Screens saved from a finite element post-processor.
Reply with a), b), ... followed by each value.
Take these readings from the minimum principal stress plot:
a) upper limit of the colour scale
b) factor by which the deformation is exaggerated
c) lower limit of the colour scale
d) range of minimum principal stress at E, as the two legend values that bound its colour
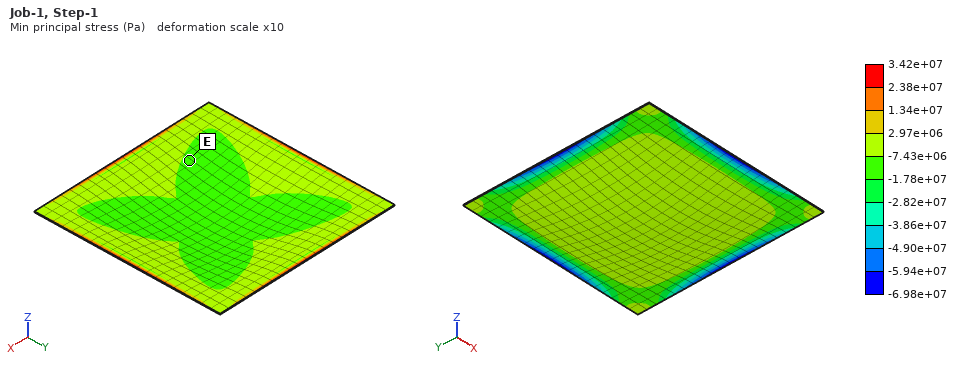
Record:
a) 3.42e+07 Pa
b) 10
c) -6.98e+07 Pa
d) -1.78e+07 to -7.43e+06 Pa
